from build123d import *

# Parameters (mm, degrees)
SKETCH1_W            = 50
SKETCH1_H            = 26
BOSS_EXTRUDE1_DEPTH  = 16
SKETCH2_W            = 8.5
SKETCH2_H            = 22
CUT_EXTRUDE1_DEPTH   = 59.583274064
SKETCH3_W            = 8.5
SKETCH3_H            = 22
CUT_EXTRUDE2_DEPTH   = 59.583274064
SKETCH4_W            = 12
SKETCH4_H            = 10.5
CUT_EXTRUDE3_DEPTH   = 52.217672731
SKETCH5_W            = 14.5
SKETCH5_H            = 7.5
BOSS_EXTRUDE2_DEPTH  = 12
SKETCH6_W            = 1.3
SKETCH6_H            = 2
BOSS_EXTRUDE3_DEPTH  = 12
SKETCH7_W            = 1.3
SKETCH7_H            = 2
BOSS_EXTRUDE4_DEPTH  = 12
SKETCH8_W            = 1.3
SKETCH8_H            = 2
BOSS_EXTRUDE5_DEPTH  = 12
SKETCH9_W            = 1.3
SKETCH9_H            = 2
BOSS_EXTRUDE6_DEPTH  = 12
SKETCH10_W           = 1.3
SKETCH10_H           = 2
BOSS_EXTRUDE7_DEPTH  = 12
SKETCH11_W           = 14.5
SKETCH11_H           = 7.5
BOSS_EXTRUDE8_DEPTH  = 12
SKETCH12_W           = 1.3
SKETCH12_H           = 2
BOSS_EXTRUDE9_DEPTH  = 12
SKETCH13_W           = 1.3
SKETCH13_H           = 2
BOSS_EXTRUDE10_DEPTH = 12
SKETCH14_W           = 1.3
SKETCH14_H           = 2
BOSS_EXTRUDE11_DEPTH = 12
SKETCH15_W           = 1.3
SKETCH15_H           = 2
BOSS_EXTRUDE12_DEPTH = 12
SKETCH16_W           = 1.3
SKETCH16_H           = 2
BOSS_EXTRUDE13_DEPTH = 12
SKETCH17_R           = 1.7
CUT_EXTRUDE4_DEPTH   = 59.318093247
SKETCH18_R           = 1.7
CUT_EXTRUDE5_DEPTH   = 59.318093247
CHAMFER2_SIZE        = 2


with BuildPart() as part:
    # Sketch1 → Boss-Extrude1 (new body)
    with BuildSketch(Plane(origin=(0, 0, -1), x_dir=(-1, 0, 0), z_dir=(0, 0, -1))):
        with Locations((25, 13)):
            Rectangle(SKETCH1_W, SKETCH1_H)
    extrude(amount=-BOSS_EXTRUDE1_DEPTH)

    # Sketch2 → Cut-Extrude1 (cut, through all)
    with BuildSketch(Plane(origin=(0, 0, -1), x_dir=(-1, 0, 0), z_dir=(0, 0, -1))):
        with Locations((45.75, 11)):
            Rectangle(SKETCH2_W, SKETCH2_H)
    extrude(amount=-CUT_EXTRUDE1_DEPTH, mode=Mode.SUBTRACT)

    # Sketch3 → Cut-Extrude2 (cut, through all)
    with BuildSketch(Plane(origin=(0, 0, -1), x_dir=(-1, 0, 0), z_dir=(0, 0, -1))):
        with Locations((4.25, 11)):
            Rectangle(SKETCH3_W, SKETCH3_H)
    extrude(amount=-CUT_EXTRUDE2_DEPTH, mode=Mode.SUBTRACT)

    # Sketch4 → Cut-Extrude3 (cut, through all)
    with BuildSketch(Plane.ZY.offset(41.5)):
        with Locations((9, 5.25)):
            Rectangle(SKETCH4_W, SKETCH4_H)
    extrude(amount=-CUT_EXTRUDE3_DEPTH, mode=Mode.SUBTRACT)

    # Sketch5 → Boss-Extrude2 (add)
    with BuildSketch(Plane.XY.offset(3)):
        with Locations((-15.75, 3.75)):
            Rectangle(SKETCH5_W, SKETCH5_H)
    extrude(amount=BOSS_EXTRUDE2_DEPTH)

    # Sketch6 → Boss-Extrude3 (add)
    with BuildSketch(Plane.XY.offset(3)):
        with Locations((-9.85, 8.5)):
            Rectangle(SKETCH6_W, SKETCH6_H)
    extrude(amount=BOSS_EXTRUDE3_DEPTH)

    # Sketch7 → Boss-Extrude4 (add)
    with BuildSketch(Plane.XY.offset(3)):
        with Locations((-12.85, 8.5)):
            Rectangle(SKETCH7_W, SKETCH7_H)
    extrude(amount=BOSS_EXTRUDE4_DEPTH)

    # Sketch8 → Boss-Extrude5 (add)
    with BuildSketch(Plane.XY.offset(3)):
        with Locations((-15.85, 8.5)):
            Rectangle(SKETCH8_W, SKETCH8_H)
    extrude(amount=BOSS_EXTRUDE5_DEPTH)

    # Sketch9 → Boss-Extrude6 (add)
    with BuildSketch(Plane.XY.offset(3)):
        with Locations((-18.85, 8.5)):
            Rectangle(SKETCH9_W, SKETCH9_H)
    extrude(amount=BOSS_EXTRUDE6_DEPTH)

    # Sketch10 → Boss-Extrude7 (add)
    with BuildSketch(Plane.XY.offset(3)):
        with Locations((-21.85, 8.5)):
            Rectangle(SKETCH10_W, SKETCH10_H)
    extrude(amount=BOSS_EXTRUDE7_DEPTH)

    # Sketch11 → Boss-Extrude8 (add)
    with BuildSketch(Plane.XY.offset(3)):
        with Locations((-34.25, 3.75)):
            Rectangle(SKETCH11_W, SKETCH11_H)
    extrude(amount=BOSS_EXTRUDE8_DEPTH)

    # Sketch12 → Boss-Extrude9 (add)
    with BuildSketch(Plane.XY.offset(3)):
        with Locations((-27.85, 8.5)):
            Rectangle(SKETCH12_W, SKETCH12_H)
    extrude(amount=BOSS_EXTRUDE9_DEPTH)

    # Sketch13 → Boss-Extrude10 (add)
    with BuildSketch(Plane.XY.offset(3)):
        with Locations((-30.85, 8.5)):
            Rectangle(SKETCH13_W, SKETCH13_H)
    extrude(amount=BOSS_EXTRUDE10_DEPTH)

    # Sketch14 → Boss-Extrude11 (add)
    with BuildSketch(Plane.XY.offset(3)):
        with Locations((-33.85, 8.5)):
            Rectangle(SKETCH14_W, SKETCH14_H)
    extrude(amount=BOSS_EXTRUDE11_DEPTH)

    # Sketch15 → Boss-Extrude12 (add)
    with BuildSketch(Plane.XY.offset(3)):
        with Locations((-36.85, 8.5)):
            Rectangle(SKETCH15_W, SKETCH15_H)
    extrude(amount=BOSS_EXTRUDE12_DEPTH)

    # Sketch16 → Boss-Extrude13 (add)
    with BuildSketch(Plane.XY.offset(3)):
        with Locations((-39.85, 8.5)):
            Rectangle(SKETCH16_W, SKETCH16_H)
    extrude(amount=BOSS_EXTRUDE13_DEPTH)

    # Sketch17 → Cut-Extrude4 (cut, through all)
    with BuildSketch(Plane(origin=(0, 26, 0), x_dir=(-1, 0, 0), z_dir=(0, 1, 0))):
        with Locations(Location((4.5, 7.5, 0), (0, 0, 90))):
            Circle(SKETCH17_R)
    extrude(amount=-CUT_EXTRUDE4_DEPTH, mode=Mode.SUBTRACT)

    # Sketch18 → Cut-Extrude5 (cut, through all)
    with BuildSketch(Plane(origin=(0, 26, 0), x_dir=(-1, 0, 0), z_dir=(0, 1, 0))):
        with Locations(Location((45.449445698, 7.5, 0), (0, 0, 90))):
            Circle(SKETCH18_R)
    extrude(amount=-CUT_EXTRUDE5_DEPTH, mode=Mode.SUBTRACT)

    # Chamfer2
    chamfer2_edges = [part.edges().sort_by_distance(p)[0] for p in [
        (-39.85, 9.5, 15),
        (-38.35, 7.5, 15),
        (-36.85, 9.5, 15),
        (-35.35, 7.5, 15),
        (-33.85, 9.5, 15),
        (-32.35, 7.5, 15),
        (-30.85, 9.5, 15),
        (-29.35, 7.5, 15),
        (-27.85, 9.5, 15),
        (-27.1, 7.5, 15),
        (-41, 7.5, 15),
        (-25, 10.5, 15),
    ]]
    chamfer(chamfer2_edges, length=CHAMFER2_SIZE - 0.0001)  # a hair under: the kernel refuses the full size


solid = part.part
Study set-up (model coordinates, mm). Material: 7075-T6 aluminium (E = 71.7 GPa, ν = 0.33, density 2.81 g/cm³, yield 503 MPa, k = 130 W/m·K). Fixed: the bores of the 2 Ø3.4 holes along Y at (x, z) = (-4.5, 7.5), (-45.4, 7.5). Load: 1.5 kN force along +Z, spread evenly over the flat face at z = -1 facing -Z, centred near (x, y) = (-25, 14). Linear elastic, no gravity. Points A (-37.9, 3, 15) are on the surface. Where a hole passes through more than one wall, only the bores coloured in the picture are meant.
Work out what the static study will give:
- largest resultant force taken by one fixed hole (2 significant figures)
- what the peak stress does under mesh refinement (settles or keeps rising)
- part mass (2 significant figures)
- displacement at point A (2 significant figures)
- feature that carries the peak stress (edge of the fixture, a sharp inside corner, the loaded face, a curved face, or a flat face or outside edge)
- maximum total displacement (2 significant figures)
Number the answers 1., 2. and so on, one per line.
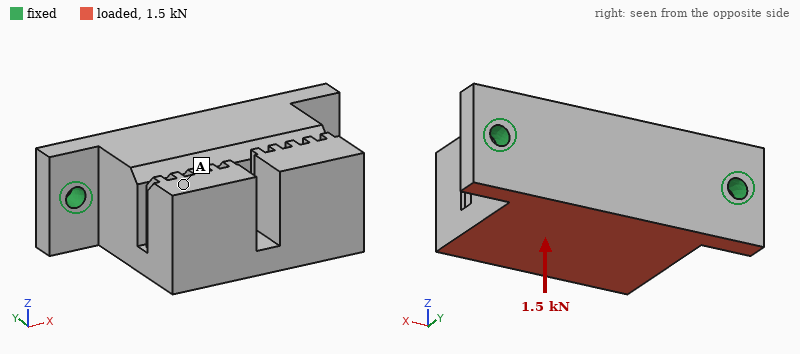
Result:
1. 750 N
2. keeps rising
3. 38 g
4. 0.12 mm
5. edge of the fixture
6. 0.14 mm
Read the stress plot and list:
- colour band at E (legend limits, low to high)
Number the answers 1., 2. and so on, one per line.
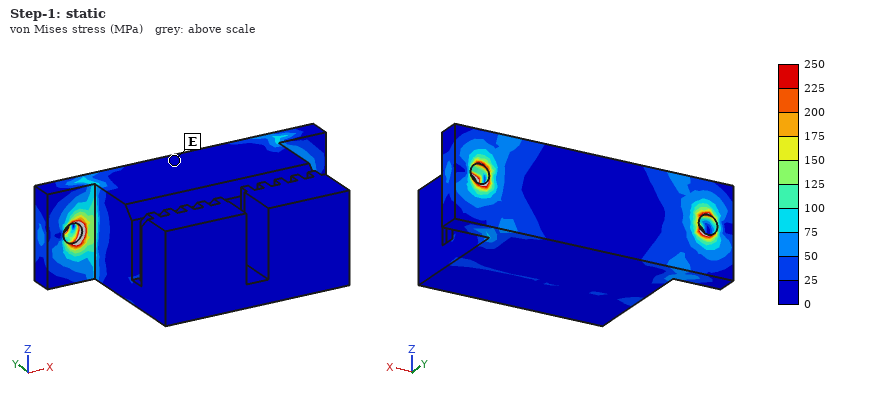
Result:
1. 0 to 25 MPa
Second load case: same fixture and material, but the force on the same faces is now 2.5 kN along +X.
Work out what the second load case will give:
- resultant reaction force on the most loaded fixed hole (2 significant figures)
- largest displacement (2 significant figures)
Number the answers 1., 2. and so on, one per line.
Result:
1. 1.5 kN
2. 18 µm
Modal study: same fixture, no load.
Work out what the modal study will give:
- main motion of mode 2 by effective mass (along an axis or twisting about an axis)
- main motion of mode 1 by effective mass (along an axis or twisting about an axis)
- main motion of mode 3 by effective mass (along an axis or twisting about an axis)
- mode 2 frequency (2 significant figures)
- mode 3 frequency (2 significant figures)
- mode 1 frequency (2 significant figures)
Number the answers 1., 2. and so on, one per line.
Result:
1. along Y
2. along Z
3. along X
4. 8700 Hz
5. 9800 Hz
6. 3400 Hz
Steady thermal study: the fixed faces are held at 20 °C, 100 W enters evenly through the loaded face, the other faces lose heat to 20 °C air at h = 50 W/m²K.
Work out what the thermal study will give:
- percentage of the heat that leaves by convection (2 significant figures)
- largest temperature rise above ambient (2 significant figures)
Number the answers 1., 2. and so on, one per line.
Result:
1. 11 %
2. 67 K
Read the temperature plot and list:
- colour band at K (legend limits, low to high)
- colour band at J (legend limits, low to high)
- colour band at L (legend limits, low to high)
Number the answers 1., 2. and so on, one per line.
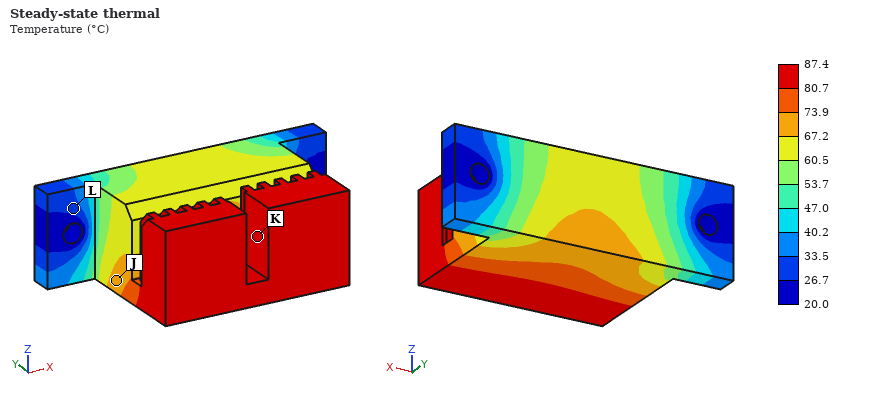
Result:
1. 80.7 to 87.4 °C
2. 67.2 to 73.9 °C
3. 26.7 to 33.5 °C
